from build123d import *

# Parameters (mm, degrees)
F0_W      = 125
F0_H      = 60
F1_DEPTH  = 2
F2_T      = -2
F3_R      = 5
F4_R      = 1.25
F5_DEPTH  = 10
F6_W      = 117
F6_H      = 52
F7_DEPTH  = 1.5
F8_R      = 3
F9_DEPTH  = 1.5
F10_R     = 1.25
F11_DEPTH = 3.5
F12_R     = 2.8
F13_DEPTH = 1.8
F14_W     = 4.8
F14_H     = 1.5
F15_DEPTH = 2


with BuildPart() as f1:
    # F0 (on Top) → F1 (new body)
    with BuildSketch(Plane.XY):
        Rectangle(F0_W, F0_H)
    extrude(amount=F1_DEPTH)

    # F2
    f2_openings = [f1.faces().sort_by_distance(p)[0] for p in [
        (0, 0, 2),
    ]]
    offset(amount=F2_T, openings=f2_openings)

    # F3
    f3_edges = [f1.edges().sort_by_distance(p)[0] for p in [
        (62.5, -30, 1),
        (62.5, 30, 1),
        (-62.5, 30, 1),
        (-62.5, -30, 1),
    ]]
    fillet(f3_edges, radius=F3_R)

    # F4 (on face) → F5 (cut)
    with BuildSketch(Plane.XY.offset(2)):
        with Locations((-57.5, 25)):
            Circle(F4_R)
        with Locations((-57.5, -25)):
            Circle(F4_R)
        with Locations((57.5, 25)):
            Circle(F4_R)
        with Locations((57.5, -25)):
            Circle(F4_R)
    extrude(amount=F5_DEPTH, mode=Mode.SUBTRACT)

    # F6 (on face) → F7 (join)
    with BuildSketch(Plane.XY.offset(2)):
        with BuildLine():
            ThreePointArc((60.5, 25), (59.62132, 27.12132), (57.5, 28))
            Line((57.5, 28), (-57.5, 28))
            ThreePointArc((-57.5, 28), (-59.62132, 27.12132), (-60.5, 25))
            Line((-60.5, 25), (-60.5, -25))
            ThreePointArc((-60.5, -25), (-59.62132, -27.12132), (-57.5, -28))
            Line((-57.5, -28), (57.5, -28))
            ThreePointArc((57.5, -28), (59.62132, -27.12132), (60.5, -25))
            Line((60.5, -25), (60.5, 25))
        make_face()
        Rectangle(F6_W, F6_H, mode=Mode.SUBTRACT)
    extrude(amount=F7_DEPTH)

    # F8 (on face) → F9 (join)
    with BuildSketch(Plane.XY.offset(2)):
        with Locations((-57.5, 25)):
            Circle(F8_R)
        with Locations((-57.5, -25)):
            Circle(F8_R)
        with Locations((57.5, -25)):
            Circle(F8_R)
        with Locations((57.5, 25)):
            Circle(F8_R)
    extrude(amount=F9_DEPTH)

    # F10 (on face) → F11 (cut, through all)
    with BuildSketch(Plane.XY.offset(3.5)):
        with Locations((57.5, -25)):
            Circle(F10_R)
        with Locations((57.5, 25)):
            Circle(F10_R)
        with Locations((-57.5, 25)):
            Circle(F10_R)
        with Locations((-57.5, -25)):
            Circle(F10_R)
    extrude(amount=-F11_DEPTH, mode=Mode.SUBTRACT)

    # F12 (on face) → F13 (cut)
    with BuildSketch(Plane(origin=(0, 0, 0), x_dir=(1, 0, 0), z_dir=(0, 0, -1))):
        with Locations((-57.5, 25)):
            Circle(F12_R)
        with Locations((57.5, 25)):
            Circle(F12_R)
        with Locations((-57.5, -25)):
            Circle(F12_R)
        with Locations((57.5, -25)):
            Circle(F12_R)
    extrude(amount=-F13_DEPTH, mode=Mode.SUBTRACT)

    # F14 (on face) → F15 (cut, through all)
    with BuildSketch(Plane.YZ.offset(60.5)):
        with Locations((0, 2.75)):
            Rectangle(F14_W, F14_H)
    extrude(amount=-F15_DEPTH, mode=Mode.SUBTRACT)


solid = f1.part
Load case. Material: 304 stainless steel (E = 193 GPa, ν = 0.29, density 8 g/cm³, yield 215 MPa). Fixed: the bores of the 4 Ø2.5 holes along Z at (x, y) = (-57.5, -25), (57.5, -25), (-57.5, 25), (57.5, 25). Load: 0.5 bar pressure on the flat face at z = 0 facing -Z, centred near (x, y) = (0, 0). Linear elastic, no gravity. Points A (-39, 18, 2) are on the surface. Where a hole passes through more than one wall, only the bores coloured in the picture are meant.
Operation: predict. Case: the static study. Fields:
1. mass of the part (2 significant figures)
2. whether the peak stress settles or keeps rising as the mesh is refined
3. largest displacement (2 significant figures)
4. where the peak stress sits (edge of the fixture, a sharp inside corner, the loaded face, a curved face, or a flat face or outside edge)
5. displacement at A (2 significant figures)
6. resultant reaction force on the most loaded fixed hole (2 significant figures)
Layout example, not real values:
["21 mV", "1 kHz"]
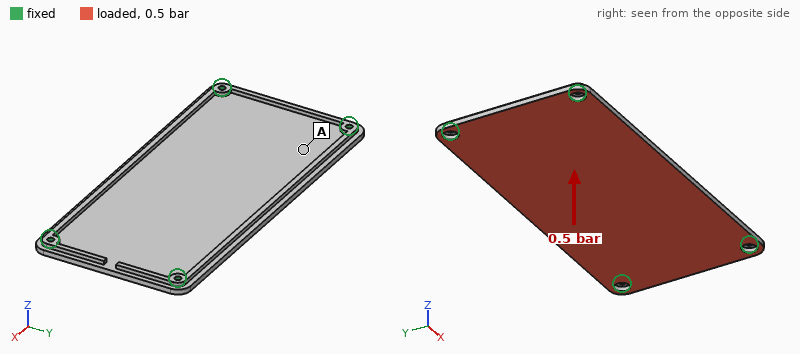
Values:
["130 g", "keeps rising", "0.17 mm", "edge of the fixture", "0.061 mm", "350 N"]
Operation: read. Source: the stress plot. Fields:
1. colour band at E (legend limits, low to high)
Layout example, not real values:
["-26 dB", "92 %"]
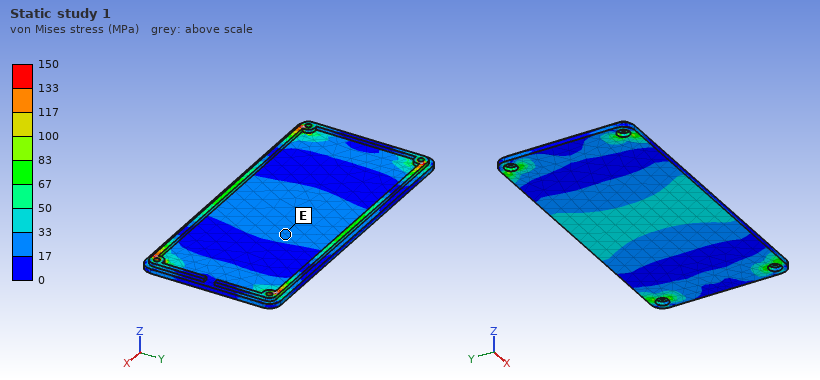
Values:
["17 to 33 MPa"]
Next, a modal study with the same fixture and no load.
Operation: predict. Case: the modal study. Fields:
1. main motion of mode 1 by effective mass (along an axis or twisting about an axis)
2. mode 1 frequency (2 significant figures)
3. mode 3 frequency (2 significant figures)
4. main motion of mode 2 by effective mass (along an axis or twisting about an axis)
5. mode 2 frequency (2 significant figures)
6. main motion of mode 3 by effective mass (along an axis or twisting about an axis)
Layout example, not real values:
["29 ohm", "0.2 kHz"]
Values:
["along Z", "770 Hz", "2000 Hz", "twisting about X", "1300 Hz", "twisting about Y"]
